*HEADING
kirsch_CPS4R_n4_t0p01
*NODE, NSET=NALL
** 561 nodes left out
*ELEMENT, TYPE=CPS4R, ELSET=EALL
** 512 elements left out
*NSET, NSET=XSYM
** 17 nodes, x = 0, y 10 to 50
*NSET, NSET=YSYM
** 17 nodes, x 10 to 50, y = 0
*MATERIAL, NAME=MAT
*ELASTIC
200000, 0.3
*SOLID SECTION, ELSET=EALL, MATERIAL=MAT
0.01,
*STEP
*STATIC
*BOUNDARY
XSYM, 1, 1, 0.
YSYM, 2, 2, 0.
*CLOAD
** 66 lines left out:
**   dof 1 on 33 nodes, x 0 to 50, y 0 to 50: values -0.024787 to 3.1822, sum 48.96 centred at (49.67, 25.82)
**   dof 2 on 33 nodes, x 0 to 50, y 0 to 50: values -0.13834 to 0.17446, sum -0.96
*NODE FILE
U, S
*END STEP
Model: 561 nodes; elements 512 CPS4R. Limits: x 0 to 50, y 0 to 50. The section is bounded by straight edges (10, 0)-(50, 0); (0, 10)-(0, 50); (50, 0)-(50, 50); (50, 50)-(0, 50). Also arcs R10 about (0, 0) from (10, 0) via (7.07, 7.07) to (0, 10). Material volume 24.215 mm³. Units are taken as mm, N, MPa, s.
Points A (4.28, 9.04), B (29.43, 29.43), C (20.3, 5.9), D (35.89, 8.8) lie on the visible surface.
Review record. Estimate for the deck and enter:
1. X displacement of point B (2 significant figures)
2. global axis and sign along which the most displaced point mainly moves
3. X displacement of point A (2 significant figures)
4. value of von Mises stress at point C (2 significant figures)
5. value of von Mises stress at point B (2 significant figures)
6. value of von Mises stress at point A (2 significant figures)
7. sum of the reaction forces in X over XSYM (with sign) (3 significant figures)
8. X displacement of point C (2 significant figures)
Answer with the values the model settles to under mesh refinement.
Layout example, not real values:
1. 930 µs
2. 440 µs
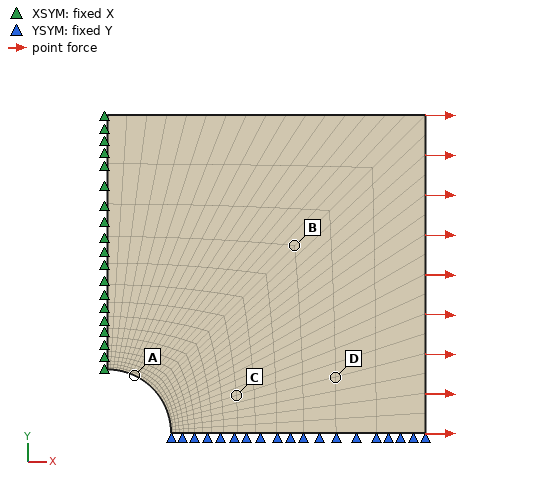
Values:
1. 0.016 mm
2. +X
3. 0.0064 mm
4. 75 MPa
5. 110 MPa
6. 230 MPa
7. -49.0 N
8. 0.015 mm
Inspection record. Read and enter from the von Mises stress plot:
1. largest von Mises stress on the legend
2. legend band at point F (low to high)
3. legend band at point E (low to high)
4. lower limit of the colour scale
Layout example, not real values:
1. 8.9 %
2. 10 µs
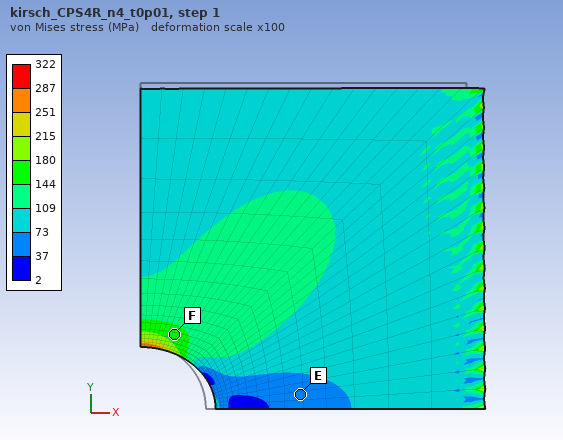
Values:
1. 322 MPa
2. 144 to 180 MPa
3. 37 to 73 MPa
4. 2 MPa
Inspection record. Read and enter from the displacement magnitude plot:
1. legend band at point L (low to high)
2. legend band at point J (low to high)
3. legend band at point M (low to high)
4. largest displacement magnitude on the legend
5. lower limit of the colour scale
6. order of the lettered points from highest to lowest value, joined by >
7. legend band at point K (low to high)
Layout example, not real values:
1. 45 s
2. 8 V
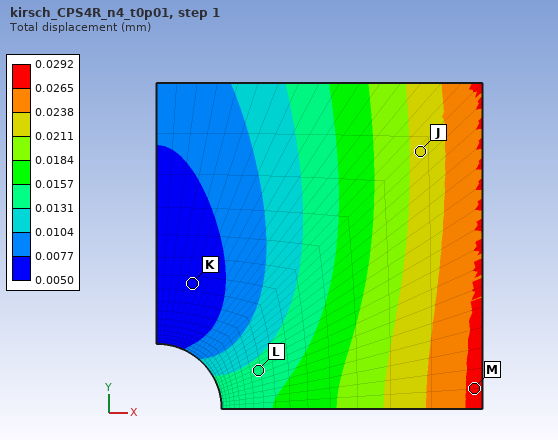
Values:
1. 0.0131 to 0.0157 mm
2. 0.0211 to 0.0238 mm
3. 0.0265 to 0.0292 mm
4. 0.0292 mm
5. 0.0050 mm
6. M > J > L > K
7. 0.0050 to 0.0077 mm
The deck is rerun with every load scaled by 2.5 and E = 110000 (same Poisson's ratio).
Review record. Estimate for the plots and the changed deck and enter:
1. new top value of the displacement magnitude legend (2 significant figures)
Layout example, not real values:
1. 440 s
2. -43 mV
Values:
1. 0.13 mm
